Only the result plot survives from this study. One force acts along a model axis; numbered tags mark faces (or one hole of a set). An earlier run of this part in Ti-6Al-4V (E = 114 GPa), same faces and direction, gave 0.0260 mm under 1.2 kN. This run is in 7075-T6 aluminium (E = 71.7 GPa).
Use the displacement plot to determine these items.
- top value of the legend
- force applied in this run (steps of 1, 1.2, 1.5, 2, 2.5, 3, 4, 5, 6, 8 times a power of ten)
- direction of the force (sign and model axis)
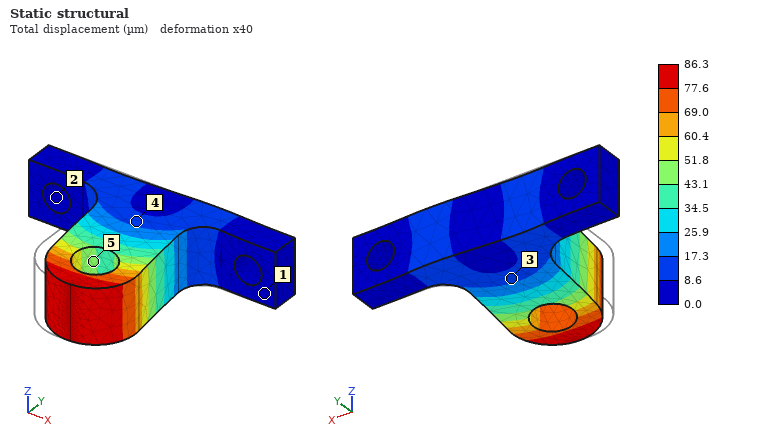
86.3 µm
2.5 kN
+X
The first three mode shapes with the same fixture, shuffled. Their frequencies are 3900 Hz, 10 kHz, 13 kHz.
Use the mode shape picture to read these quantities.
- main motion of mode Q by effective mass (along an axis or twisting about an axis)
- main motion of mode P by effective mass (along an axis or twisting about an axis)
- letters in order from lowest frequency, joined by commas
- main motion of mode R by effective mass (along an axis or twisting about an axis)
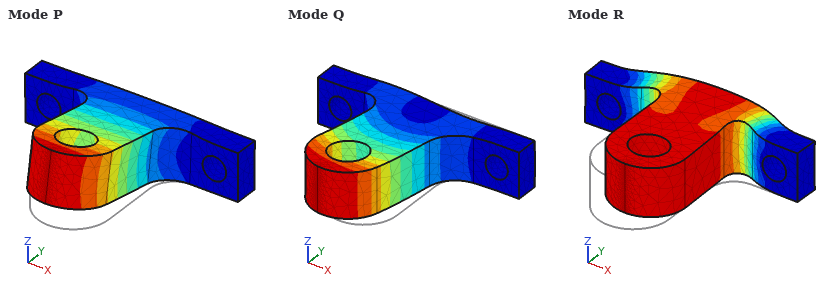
along X
along Z
P, Q, R
along Y
